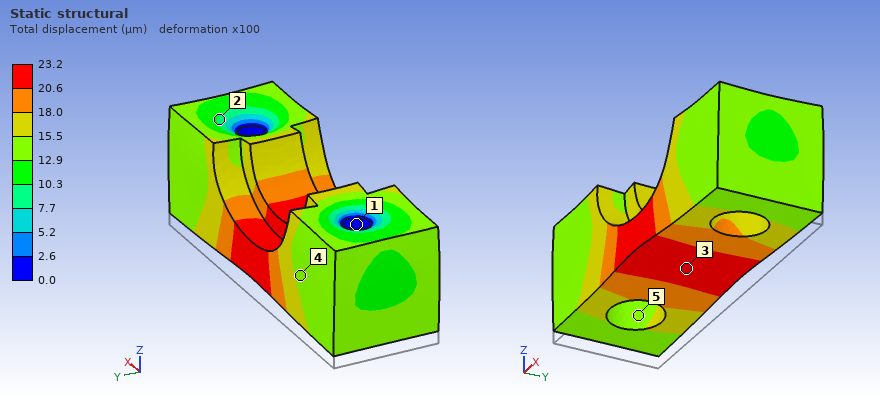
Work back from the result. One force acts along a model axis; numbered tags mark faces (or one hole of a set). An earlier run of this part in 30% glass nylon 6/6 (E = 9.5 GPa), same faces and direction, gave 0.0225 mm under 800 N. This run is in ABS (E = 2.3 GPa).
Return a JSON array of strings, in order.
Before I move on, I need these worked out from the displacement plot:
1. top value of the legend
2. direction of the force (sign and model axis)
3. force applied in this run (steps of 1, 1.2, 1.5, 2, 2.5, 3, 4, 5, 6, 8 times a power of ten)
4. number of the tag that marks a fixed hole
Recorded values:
["23.2 µm", "+Z", "200 N", "1"]
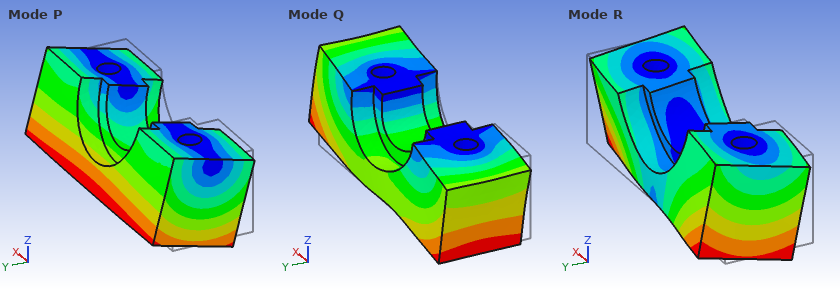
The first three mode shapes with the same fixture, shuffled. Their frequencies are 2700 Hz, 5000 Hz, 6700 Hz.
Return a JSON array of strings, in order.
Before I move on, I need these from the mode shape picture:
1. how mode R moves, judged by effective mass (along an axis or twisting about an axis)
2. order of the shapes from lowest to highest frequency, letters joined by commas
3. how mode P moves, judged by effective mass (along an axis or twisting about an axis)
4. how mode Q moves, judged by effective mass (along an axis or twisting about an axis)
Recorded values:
["twisting about Z", "P, R, Q", "along Y", "along X"]
